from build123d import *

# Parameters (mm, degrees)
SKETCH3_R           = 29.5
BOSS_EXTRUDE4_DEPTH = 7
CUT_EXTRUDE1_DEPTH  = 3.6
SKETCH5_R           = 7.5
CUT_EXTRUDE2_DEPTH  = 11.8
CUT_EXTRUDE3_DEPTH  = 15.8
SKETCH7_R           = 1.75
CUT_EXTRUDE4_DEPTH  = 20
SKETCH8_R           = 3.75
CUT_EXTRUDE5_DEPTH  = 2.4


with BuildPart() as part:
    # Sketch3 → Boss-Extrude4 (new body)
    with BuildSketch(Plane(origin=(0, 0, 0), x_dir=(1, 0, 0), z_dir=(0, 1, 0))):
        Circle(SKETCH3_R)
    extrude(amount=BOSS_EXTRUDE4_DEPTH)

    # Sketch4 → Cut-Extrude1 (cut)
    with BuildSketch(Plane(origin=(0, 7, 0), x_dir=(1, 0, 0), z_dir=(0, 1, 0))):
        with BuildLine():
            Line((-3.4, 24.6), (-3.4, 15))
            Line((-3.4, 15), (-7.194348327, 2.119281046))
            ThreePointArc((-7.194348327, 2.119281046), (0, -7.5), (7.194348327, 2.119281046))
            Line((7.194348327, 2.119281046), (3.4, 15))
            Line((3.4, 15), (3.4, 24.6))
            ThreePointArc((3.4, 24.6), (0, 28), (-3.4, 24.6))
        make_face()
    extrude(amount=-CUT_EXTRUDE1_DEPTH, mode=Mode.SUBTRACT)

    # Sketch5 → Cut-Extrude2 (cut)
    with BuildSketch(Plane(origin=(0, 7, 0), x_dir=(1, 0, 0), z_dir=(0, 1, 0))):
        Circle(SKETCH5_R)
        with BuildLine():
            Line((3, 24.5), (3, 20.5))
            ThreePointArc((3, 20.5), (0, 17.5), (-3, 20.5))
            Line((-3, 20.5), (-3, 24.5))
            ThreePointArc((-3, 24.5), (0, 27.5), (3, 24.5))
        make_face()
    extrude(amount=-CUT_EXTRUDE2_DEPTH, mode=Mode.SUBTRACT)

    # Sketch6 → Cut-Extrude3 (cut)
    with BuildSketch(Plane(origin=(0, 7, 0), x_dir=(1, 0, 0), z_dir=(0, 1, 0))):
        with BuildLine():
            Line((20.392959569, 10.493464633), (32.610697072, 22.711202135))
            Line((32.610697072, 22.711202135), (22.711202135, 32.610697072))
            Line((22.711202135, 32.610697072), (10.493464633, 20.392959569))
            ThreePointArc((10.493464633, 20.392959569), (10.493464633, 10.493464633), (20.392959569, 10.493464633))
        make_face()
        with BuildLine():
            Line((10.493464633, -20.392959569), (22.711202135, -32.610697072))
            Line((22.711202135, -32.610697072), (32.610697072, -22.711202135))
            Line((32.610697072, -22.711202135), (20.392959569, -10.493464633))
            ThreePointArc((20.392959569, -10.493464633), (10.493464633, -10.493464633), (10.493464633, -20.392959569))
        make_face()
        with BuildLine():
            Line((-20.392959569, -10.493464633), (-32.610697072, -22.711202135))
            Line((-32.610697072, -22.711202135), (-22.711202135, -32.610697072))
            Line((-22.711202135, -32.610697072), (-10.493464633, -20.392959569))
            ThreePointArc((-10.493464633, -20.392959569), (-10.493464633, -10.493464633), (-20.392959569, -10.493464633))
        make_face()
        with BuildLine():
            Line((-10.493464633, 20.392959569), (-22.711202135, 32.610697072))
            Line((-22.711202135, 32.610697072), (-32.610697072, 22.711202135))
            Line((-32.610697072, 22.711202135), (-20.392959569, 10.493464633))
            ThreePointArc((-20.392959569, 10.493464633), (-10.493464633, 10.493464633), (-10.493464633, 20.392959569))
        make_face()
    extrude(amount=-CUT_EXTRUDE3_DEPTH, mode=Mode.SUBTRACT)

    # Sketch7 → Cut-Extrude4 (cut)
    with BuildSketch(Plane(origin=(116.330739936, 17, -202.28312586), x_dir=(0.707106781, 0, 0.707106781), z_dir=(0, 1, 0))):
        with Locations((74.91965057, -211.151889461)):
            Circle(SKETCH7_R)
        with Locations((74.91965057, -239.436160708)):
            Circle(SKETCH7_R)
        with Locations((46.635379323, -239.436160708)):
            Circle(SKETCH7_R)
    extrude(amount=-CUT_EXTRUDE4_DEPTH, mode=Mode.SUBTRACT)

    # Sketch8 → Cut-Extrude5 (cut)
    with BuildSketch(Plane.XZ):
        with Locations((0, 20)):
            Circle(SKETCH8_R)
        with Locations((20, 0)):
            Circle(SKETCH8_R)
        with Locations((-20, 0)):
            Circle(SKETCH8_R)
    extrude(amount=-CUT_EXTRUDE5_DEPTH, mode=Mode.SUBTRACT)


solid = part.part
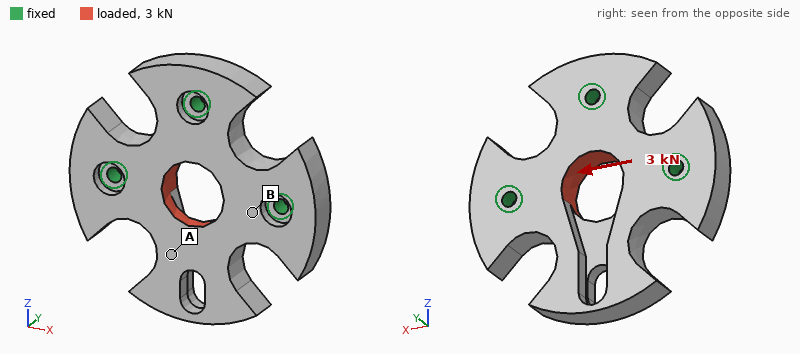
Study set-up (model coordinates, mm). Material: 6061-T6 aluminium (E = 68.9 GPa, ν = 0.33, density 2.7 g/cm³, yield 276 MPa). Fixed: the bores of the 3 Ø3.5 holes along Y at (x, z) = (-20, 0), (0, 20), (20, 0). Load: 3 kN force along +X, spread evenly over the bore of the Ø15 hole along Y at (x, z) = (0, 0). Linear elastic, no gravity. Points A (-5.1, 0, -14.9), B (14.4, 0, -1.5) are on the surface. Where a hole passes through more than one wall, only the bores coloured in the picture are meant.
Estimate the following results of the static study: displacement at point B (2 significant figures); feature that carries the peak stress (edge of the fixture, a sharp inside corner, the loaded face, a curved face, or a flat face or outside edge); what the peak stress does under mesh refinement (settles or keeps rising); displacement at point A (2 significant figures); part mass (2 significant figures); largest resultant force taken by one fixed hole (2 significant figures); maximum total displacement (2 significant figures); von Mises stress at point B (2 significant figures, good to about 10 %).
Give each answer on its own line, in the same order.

2.6 µm
edge of the fixture
keeps rising
3.0 µm
31 g
1.3 kN
5.8 µm
7.2 MPa
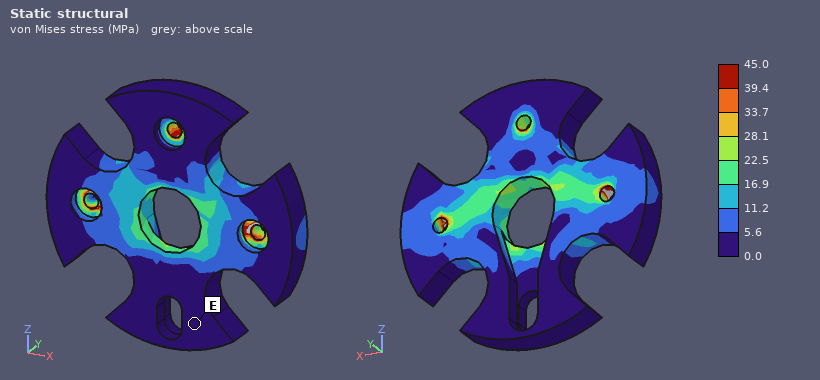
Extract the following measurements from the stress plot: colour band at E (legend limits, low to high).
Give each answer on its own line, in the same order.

0.0 to 5.6 MPa
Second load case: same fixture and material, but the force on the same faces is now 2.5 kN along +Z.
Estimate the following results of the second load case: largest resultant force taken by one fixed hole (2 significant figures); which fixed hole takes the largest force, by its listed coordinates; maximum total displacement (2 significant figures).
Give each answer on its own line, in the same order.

1.5 kN
(0, 20)
21 µm
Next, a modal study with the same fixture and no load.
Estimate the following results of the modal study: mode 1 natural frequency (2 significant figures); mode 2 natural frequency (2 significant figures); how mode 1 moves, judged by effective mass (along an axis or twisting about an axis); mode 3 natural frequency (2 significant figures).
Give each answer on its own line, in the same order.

4500 Hz
9900 Hz
along Y
13 kHz
